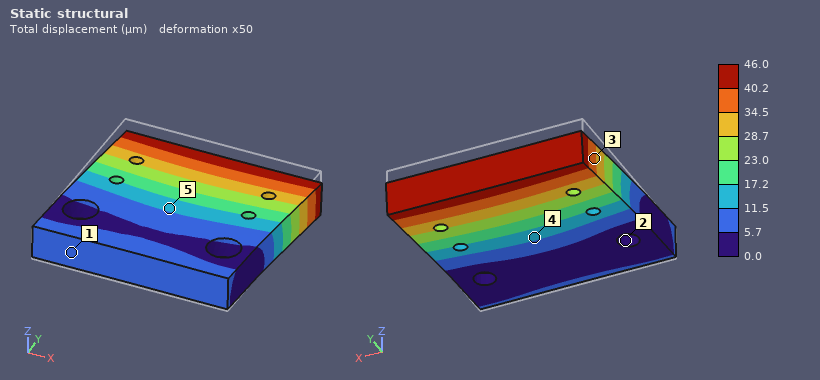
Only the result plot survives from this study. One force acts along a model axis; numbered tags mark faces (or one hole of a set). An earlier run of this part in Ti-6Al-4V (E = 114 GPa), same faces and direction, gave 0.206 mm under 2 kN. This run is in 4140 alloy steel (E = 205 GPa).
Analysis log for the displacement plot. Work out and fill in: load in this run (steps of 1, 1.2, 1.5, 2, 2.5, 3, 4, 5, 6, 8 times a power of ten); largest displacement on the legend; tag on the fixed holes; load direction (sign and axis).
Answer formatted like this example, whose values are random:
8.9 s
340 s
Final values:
800 N
46.0 µm
2
-Z
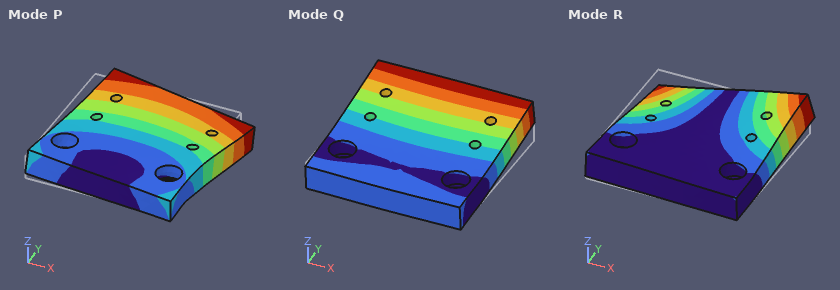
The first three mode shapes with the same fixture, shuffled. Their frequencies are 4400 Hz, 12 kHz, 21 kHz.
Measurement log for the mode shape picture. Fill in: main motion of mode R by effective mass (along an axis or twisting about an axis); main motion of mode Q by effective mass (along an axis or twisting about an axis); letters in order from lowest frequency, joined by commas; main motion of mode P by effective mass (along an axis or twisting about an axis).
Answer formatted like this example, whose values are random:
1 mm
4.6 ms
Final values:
twisting about Y
along Z
Q, R, P
along X
